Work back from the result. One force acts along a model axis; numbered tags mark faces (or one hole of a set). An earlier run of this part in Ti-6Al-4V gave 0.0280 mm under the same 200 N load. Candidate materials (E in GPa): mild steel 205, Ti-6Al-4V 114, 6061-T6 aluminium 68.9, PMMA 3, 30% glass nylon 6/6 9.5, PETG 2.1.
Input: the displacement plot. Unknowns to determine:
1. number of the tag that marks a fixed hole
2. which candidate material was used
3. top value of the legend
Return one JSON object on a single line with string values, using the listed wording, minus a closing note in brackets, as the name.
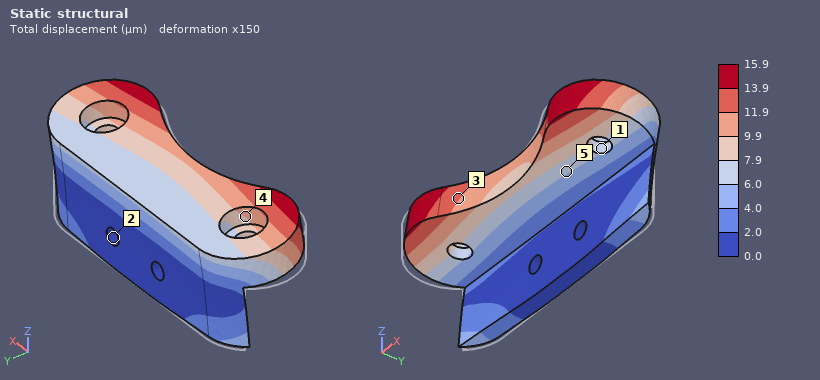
{"number of the tag that marks a fixed hole": "2", "which candidate material was used": "mild steel", "top value of the legend": "15.9 µm"}
